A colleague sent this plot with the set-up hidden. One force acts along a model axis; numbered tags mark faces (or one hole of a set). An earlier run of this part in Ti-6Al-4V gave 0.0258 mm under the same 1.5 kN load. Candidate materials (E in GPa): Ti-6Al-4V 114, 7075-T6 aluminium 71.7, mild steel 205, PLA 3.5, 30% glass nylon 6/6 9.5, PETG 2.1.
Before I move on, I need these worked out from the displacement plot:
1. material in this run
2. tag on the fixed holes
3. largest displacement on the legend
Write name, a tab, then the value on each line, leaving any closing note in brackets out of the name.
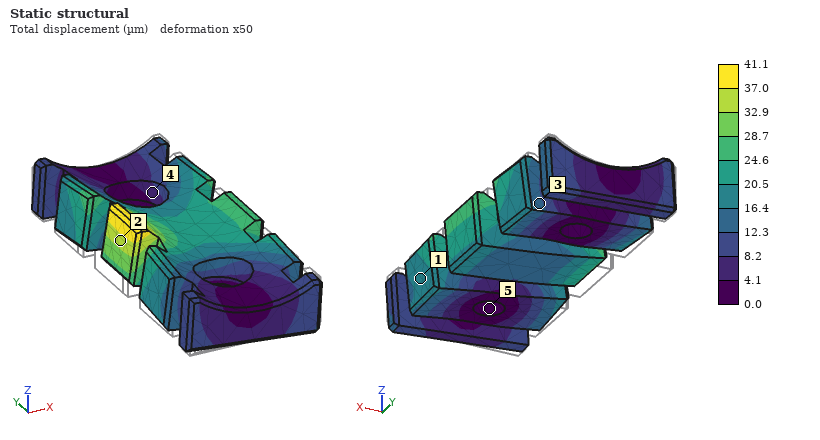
material in this run	7075-T6 aluminium
tag on the fixed holes	5
largest displacement on the legend	41.1 µm
